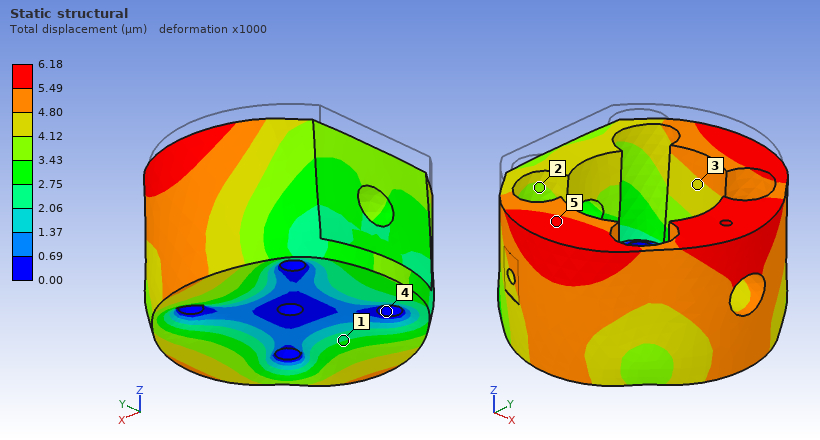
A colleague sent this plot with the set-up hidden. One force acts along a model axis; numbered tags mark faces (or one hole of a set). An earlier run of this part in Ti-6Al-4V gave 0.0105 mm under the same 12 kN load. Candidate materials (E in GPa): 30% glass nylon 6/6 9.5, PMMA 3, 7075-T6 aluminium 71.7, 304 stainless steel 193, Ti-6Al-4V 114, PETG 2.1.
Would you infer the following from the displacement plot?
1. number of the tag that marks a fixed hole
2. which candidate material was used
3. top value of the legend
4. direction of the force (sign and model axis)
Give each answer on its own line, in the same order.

4
304 stainless steel
6.18 µm
-Z
